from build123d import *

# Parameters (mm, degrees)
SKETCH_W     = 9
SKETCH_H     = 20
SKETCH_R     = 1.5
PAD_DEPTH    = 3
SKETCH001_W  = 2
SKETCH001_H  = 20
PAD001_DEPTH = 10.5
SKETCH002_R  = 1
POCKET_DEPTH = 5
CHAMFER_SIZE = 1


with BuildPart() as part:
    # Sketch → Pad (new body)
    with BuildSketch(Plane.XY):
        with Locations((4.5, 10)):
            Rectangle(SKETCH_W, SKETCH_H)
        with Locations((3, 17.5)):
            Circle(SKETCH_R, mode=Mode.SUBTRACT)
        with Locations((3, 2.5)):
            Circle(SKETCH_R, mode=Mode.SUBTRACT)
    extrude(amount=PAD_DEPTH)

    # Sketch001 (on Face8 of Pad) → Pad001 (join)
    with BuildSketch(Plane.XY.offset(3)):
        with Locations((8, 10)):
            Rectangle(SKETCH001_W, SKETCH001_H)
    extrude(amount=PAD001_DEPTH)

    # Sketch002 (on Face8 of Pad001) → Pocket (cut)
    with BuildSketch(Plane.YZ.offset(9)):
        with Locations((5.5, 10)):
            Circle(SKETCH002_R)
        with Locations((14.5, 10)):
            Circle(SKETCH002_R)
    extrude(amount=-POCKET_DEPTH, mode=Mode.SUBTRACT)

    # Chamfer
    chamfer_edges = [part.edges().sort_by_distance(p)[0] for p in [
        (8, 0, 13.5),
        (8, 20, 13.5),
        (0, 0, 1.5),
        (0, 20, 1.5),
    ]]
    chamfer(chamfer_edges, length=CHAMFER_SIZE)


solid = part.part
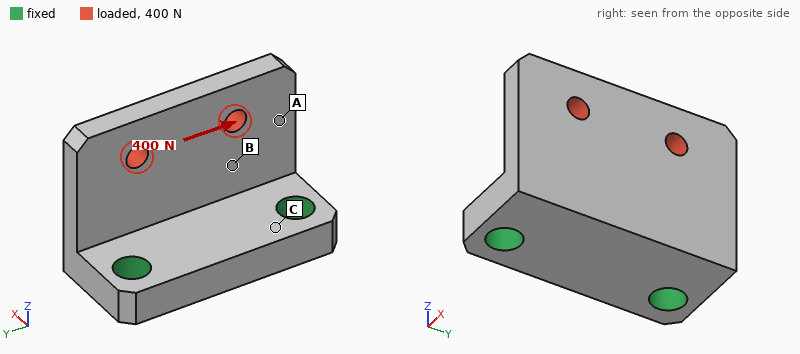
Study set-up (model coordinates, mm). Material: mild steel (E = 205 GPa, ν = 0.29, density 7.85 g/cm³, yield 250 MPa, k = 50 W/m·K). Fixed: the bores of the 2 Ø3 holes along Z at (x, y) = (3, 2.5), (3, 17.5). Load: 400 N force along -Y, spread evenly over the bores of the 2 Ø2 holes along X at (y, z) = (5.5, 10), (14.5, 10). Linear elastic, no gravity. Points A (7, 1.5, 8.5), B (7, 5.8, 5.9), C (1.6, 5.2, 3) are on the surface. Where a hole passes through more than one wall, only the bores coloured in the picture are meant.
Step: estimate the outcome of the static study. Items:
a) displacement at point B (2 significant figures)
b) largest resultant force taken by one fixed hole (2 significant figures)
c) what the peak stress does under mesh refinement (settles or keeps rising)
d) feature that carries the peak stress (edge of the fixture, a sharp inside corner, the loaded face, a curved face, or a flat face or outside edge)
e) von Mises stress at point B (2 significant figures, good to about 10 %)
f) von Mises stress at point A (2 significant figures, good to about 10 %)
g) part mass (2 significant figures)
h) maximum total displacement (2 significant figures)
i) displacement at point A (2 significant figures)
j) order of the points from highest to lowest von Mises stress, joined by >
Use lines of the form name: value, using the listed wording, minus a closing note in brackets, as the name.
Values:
displacement at point B: 2.4 µm
largest resultant force taken by one fixed hole: 310 N
what the peak stress does under mesh refinement: keeps rising
feature that carries the peak stress: edge of the fixture
von Mises stress at point B: 31 MPa
von Mises stress at point A: 16 MPa
part mass: 7.1 g
maximum total displacement: 6.2 µm
displacement at point A: 4.4 µm
order of the points from highest to lowest von Mises stress, joined by >: B > A > C
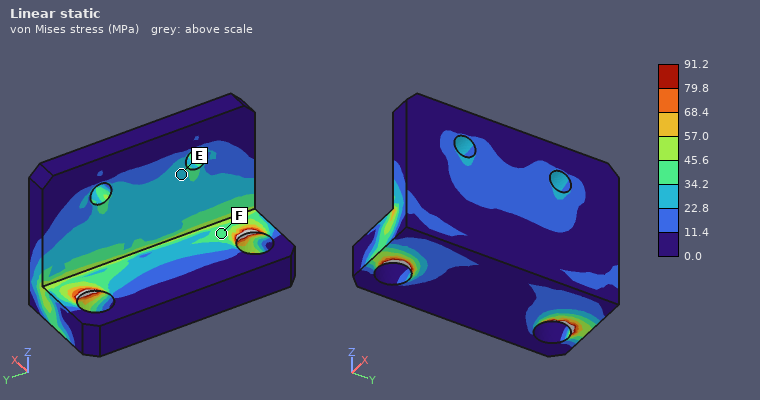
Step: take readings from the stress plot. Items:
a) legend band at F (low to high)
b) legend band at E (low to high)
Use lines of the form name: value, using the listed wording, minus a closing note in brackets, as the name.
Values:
legend band at F: 34.2 to 45.6 MPa
legend band at E: 22.8 to 34.2 MPa
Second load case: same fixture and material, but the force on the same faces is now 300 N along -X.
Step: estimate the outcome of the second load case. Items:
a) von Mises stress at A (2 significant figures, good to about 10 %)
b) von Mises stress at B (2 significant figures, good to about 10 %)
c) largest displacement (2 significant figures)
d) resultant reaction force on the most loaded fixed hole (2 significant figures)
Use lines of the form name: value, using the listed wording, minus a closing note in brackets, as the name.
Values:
von Mises stress at A: 39 MPa
von Mises stress at B: 90 MPa
largest displacement: 46 µm
resultant reaction force on the most loaded fixed hole: 160 N
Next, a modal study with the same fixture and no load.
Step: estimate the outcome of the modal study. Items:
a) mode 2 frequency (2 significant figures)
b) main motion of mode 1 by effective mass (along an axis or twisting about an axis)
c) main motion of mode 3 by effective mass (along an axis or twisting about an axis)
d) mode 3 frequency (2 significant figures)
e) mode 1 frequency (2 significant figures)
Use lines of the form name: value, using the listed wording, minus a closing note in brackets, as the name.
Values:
mode 2 frequency: 18 kHz
main motion of mode 1 by effective mass: along X
main motion of mode 3 by effective mass: along Y
mode 3 frequency: 31 kHz
mode 1 frequency: 10 kHz
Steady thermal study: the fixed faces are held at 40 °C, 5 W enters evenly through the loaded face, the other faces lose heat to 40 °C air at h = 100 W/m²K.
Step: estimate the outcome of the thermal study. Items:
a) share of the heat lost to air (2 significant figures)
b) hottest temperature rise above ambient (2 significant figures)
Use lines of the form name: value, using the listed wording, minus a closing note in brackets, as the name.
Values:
share of the heat lost to air: 21 %
hottest temperature rise above ambient: 28 K
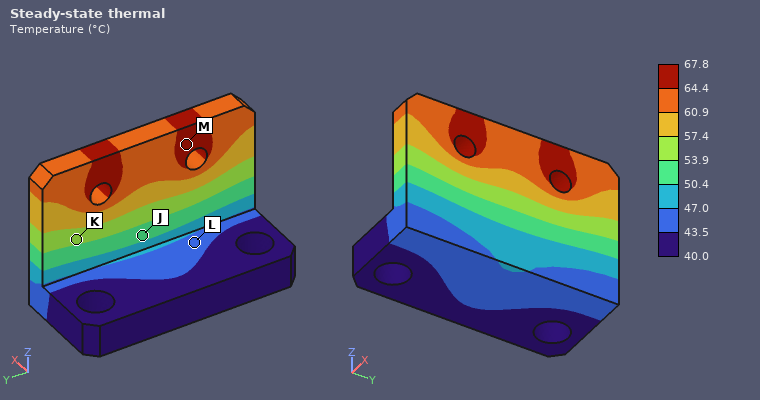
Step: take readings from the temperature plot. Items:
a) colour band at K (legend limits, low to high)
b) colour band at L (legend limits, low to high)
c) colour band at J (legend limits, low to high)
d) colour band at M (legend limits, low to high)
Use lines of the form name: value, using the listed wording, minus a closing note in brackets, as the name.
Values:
colour band at K: 53.9 to 57.4 °C
colour band at L: 43.5 to 47.0 °C
colour band at J: 50.4 to 53.9 °C
colour band at M: 64.4 to 67.8 °C
